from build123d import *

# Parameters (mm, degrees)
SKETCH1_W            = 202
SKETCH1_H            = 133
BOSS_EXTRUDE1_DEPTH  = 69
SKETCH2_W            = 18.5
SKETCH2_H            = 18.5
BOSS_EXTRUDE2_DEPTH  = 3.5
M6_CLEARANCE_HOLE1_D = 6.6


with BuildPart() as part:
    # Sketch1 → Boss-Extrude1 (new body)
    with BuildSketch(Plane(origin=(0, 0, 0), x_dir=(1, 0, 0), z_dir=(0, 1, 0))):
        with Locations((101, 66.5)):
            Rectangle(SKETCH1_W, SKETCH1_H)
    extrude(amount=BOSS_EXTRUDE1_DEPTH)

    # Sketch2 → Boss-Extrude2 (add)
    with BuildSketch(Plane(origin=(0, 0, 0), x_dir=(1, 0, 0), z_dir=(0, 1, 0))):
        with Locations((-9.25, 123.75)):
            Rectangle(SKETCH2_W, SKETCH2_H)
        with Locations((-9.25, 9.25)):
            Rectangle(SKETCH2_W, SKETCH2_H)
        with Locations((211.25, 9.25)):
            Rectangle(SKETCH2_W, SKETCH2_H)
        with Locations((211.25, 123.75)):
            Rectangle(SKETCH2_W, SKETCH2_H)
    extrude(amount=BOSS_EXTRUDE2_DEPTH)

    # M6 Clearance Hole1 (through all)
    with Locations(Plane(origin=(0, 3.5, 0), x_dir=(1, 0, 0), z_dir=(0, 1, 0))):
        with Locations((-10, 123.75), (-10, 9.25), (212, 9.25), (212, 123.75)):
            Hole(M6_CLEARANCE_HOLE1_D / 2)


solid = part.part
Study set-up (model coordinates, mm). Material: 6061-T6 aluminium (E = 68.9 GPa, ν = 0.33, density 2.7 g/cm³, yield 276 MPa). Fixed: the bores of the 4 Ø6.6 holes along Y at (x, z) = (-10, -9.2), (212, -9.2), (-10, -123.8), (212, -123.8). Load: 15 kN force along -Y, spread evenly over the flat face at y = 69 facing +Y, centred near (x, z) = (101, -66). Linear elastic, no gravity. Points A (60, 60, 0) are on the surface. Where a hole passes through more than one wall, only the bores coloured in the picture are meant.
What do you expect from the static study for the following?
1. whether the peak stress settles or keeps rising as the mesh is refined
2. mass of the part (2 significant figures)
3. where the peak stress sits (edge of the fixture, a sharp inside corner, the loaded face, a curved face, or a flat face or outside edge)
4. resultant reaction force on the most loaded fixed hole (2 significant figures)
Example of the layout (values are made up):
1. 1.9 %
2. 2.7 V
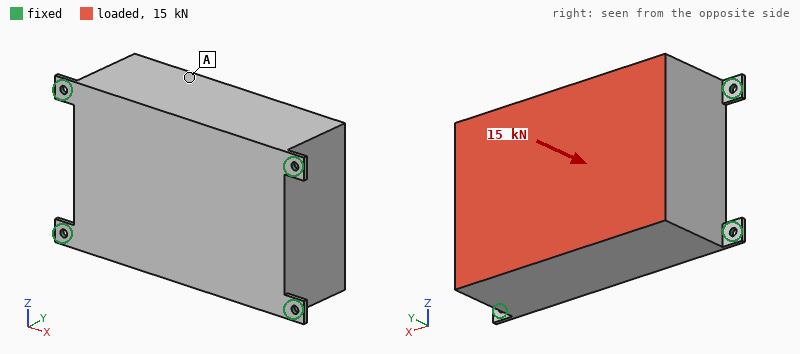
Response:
1. keeps rising
2. 5.0 kg
3. edge of the fixture
4. 4.4 kN
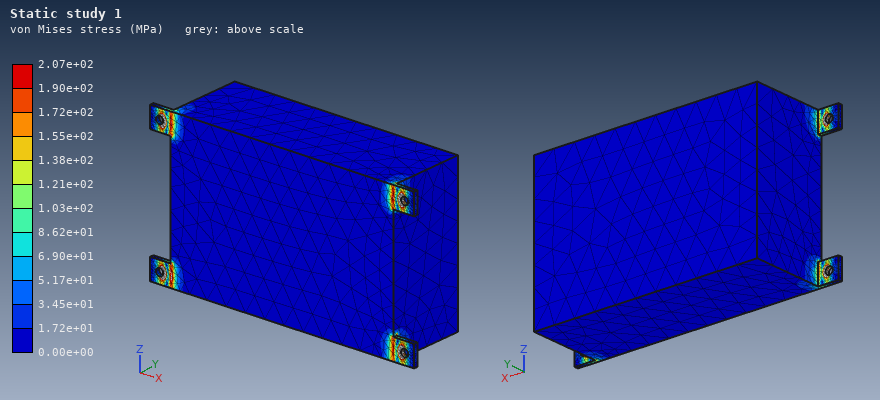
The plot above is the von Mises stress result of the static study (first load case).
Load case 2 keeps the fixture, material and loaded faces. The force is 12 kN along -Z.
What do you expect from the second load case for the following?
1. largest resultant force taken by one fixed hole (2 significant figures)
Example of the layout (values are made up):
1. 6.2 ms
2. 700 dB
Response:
1. 5.3 kN
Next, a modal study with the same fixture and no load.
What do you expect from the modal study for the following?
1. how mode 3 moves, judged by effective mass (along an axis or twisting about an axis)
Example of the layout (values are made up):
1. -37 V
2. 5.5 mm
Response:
1. along X
